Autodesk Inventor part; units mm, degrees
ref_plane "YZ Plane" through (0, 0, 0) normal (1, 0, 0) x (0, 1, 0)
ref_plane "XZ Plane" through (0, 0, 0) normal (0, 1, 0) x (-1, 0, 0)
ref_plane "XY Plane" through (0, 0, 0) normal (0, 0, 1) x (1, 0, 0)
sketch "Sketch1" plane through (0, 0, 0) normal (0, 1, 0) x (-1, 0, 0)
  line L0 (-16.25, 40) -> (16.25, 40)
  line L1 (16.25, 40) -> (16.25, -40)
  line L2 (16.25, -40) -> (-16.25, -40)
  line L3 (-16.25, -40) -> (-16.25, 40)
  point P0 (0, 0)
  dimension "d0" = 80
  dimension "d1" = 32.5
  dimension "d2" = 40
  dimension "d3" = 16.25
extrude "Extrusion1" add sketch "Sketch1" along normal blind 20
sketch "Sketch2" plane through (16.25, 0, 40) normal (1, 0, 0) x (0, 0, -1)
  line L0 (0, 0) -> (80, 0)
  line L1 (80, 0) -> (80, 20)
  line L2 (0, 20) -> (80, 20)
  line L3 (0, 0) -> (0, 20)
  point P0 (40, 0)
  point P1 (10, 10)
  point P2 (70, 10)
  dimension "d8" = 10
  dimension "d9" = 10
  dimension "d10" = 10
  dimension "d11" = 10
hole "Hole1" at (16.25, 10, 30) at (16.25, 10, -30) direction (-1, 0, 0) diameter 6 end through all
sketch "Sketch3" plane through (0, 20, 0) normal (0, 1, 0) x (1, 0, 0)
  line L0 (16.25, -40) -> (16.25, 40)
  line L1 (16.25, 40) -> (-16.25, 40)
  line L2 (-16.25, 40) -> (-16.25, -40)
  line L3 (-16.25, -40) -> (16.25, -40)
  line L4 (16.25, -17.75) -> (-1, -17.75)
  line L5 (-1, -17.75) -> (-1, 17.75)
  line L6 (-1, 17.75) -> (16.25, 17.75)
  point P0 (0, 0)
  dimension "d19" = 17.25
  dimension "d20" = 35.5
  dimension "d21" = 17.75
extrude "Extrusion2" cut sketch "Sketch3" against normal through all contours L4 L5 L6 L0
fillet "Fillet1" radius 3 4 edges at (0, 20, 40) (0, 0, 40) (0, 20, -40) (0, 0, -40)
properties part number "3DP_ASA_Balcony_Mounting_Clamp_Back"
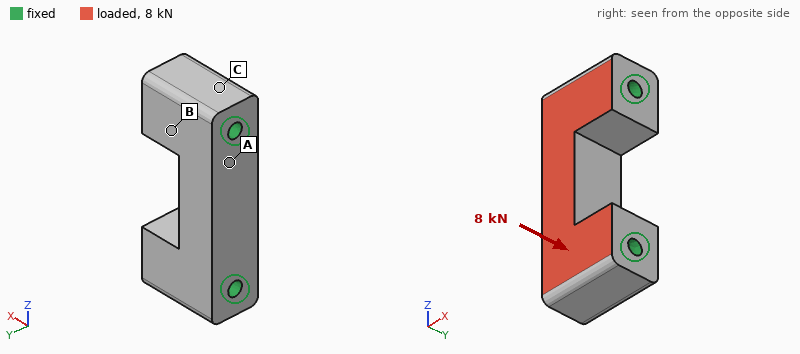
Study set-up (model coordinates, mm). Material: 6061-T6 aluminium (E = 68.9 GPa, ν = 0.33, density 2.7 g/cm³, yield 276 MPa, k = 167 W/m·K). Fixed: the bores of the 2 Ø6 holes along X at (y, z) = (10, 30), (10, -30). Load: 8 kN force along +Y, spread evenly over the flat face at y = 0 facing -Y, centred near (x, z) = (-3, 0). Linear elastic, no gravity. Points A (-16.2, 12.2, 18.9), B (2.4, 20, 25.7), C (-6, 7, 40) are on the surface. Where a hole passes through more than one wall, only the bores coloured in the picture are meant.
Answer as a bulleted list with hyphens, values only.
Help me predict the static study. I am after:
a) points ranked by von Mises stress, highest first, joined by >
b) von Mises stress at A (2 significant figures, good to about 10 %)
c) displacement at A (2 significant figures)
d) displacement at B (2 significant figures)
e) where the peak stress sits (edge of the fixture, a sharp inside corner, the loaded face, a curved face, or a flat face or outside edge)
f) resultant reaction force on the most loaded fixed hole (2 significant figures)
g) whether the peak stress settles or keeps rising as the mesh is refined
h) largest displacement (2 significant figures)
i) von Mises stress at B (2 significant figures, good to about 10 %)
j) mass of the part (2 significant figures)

- A > B > C
- 11 MPa
- 4.6 µm
- 2.2 µm
- edge of the fixture
- 4.0 kN
- keeps rising
- 9.7 µm
- 6.3 MPa
- 100 g
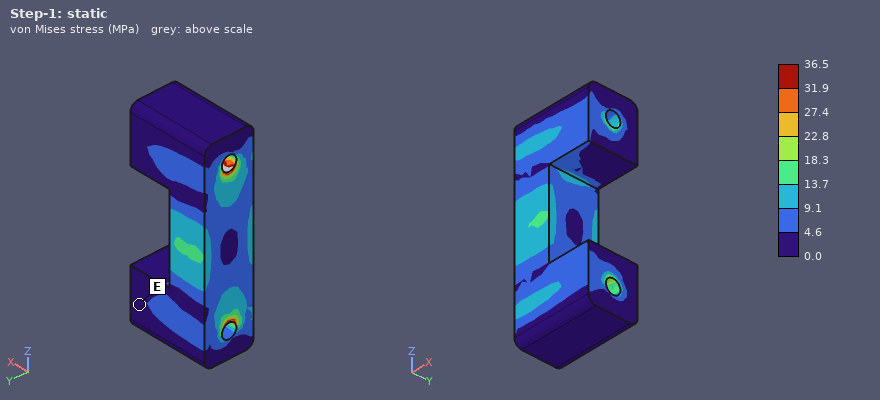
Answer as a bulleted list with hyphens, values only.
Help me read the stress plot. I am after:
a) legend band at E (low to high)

- 0.0 to 4.6 MPa
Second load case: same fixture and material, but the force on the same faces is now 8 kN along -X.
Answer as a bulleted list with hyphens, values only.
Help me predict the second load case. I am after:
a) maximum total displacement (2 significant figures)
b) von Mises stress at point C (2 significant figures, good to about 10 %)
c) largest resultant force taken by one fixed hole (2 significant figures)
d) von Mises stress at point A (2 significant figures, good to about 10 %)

- 15 µm
- 3.3 MPa
- 4.0 kN
- 13 MPa
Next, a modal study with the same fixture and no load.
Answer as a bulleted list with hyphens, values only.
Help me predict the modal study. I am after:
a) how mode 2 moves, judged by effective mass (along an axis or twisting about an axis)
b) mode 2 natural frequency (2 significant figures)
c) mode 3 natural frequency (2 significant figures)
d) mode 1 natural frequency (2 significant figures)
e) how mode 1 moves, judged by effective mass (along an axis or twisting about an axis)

- along X
- 22 kHz
- 29 kHz
- 17 kHz
- along Y
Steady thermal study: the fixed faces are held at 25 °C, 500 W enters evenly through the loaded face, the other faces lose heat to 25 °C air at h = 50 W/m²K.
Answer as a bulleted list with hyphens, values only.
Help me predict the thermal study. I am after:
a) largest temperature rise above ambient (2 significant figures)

- 45 K
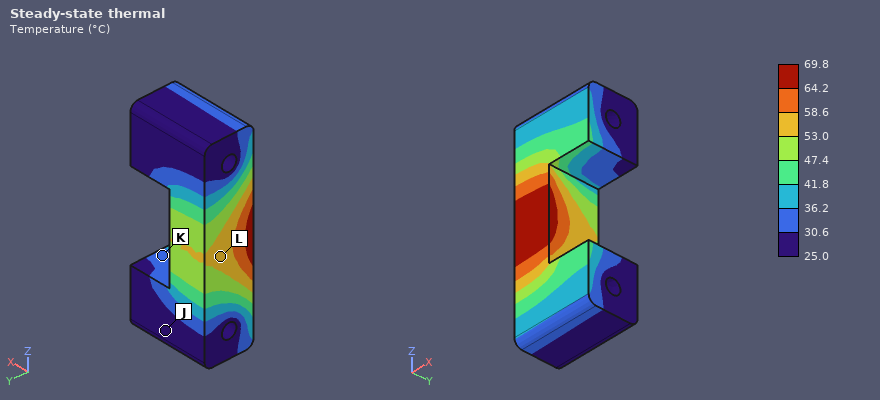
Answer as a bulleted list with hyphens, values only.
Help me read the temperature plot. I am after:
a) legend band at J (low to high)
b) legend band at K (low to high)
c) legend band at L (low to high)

- 25.0 to 30.6 °C
- 30.6 to 36.2 °C
- 53.0 to 58.6 °C
